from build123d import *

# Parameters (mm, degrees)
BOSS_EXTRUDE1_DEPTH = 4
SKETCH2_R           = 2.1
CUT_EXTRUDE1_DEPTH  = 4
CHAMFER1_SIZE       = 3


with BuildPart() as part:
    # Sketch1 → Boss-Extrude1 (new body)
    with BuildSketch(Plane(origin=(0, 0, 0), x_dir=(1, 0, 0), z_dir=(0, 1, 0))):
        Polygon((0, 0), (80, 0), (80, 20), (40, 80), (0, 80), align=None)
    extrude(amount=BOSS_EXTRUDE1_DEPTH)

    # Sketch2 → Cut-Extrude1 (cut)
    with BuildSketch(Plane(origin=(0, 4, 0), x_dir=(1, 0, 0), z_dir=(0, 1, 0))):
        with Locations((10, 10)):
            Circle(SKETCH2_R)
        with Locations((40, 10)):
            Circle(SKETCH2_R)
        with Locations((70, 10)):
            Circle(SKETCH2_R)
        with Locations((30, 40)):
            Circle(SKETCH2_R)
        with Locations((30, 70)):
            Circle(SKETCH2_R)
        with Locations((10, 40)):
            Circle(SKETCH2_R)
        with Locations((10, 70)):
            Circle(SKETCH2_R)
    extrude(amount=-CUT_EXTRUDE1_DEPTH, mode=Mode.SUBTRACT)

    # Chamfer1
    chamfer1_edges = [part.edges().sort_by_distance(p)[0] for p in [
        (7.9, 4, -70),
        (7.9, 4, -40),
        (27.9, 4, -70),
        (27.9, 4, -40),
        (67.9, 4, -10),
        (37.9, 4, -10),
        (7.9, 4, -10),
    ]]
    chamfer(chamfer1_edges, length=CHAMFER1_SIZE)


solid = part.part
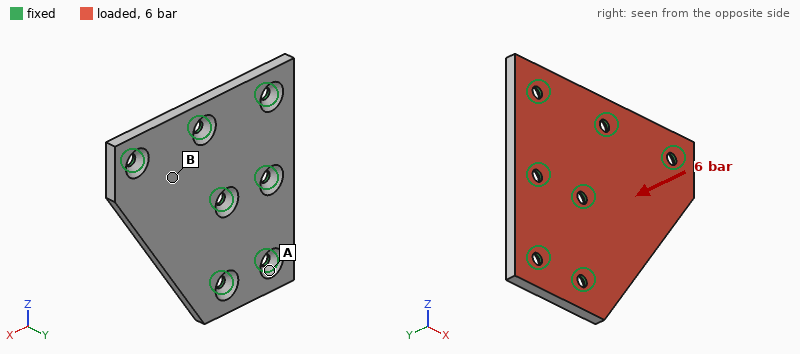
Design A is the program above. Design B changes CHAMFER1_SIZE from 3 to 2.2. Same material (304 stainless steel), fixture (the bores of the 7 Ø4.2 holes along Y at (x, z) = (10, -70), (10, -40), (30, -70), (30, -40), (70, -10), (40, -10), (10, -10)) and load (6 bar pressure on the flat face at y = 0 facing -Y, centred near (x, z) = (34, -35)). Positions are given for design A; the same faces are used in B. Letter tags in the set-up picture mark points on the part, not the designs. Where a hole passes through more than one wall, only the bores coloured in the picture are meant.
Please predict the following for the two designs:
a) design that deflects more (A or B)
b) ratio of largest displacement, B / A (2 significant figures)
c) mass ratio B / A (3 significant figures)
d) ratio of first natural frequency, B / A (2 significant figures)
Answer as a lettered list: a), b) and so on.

a) A
b) 0.88
c) 1.02
d) 1.1
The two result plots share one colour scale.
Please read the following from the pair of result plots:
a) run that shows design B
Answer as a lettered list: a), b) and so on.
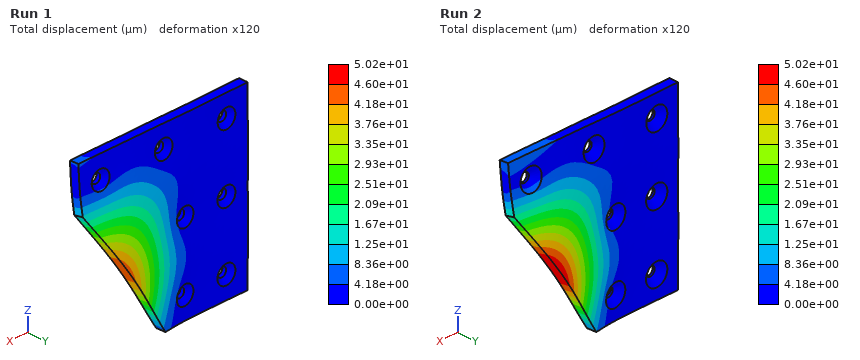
a) Run 1
